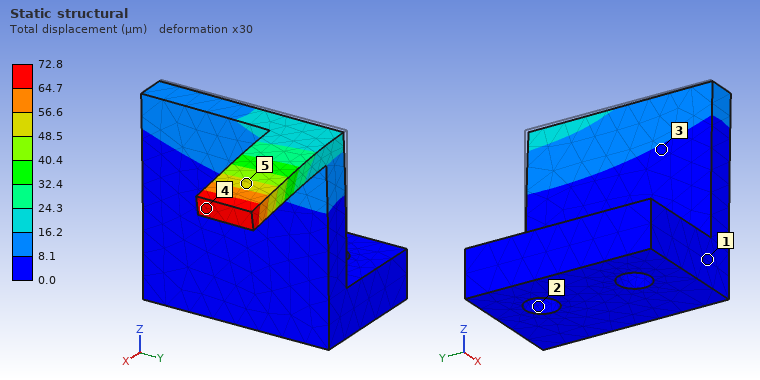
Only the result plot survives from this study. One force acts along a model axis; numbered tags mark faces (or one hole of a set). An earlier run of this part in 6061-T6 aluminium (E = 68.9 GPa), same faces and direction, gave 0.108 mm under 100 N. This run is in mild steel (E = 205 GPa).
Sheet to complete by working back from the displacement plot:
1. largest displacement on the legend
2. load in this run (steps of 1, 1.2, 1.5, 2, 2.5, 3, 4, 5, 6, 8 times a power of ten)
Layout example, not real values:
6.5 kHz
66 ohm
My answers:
72.8 µm
200 N
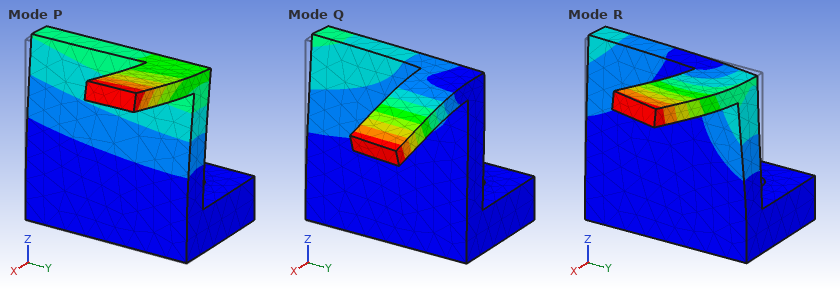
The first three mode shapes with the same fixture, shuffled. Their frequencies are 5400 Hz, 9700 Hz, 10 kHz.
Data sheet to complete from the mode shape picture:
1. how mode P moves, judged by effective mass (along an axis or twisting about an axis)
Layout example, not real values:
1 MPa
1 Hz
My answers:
along X
